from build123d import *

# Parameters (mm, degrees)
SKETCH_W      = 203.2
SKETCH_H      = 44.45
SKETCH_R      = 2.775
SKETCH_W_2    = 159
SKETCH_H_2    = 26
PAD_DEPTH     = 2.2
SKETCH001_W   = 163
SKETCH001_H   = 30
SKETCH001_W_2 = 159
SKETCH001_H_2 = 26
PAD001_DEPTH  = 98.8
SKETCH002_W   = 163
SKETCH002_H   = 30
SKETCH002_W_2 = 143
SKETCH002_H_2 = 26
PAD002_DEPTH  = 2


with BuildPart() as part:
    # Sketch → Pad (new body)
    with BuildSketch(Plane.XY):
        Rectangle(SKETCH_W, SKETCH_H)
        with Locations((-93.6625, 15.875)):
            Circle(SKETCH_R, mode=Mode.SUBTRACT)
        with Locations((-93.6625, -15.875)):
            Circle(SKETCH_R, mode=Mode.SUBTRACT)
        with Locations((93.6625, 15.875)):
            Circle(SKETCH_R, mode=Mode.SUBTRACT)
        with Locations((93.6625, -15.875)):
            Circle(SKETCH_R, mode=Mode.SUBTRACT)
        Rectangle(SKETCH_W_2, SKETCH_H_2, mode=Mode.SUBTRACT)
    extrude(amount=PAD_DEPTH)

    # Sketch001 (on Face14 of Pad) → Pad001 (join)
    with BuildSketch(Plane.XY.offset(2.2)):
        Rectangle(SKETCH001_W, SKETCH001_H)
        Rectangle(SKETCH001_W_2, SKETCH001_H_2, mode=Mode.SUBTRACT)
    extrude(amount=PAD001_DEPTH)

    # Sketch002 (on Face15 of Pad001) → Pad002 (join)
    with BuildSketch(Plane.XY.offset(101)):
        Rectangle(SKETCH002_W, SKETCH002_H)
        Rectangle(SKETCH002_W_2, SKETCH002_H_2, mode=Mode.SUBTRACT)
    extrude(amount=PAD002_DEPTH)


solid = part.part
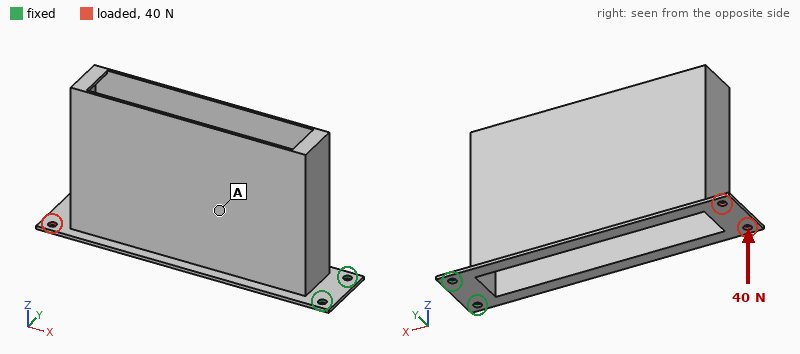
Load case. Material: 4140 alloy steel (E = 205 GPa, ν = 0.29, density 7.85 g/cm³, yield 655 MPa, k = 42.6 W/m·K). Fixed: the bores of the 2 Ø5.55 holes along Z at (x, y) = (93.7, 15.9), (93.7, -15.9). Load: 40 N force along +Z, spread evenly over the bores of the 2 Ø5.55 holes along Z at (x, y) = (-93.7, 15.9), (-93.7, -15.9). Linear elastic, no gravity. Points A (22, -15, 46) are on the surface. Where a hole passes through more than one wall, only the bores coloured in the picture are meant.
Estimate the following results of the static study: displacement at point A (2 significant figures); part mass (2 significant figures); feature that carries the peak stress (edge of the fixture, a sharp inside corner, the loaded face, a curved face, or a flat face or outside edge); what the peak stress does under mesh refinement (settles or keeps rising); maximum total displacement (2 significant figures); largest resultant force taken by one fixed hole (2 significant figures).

0.98 mm
690 g
edge of the fixture
keeps rising
2.5 mm
58 N
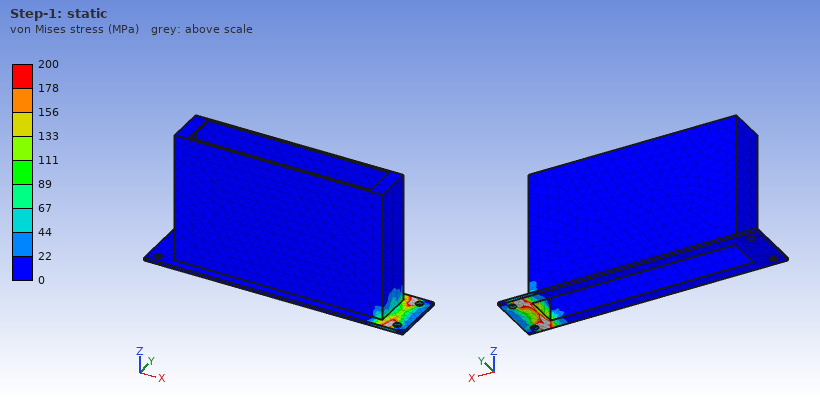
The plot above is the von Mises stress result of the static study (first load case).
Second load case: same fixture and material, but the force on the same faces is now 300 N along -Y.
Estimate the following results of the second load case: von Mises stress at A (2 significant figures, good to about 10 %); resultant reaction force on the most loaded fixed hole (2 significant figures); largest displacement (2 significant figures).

20 MPa
1.6 kN
1.2 mm
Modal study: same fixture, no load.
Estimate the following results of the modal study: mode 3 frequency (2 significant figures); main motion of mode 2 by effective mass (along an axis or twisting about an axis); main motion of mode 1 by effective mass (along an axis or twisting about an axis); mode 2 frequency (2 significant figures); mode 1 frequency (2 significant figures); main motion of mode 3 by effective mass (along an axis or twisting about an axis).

300 Hz
along Y
along Z
140 Hz
39 Hz
twisting about X
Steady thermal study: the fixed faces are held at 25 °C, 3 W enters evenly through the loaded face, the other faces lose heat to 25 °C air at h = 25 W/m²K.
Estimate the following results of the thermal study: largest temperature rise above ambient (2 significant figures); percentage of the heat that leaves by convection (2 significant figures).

23 K
100 %
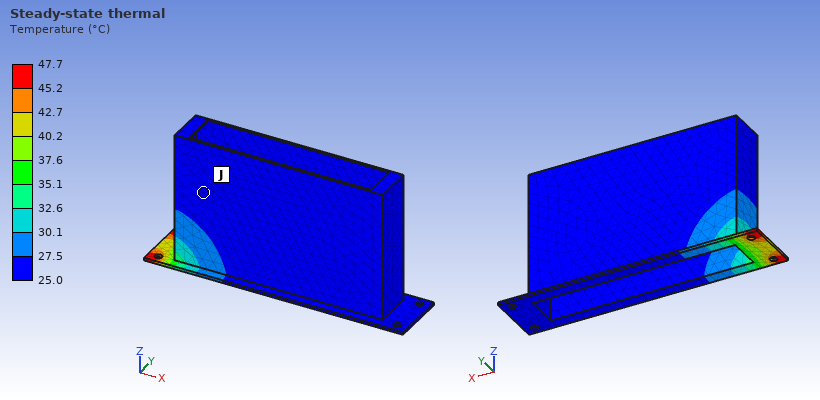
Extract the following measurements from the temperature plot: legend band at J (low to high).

25.0 to 27.5 °C
